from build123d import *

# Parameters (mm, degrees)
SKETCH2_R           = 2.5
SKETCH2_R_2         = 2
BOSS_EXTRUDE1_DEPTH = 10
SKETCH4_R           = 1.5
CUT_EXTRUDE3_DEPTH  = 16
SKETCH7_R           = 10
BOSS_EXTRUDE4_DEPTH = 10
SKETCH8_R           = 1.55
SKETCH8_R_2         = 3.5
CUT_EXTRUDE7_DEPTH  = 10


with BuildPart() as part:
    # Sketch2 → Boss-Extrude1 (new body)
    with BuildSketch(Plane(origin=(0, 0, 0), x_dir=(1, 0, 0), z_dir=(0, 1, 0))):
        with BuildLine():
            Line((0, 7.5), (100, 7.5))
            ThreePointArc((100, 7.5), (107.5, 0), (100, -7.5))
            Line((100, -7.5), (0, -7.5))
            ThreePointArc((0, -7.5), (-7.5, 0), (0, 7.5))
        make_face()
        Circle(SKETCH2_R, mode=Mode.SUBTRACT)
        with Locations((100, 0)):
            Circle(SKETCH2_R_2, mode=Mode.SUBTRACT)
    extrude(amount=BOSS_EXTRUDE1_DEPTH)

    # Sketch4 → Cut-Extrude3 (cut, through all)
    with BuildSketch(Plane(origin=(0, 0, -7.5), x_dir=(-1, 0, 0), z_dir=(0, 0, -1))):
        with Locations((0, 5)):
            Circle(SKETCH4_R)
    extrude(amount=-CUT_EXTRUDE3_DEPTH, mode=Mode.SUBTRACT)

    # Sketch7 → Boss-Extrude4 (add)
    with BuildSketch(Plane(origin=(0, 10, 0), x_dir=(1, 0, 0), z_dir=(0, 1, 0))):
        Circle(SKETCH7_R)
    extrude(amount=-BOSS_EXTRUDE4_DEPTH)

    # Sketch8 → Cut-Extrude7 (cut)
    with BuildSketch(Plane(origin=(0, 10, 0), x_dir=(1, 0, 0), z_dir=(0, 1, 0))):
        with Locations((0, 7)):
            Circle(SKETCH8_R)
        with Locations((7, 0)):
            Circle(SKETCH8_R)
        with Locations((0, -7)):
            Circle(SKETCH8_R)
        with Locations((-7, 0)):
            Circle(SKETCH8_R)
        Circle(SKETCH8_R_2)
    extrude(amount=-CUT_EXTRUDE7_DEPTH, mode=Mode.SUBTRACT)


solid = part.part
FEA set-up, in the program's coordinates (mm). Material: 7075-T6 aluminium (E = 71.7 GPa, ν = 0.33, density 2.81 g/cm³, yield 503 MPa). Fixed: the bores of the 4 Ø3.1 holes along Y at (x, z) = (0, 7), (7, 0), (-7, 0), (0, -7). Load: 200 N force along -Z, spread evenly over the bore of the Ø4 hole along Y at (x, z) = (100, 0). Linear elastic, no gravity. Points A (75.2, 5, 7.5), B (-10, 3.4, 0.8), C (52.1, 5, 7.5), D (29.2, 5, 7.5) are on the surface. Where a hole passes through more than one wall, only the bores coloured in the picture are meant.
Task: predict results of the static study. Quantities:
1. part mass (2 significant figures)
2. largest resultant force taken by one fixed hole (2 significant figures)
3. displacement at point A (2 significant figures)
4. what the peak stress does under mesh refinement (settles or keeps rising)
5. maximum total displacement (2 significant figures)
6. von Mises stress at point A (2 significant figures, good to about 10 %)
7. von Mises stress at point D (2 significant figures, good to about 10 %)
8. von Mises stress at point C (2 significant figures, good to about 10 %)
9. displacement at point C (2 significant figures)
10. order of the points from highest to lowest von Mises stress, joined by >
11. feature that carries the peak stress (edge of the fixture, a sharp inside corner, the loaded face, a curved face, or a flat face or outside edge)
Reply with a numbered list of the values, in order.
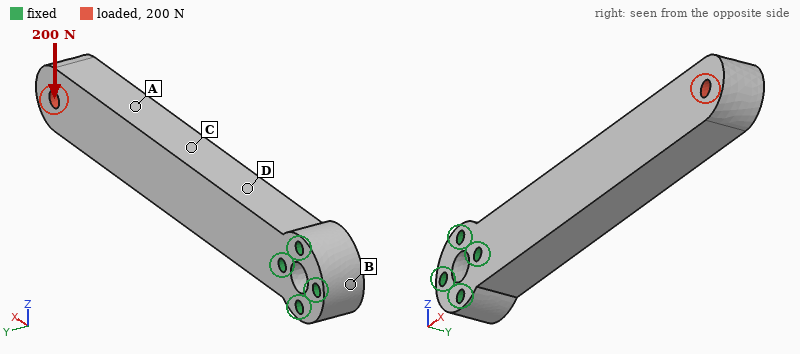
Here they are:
1. 47 g
2. 1.1 kN
3. 0.19 mm
4. keeps rising
5. 0.34 mm
6. 13 MPa
7. 38 MPa
8. 26 MPa
9. 0.10 mm
10. D > C > A > B
11. a sharp inside corner
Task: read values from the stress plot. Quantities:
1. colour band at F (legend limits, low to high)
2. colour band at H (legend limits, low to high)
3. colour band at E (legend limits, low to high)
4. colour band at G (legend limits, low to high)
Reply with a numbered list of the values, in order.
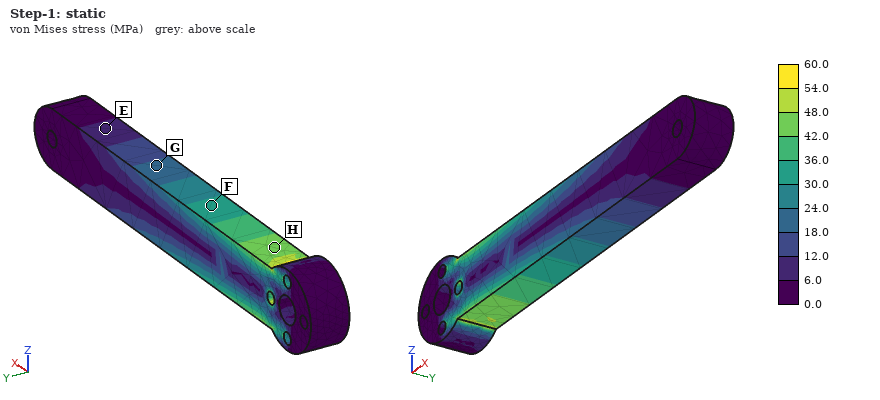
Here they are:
1. 30.0 to 36.0 MPa
2. 42.0 to 48.0 MPa
3. 6.0 to 12.0 MPa
4. 18.0 to 24.0 MPa
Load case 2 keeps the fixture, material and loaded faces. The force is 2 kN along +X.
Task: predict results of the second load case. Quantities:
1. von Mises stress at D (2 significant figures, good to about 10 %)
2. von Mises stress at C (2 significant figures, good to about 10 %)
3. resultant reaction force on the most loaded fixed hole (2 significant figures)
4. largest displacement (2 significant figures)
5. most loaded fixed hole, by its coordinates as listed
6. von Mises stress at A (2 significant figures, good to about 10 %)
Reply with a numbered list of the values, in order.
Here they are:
1. 13 MPa
2. 13 MPa
3. 1.3 kN
4. 19 µm
5. (7, 0)
6. 13 MPa
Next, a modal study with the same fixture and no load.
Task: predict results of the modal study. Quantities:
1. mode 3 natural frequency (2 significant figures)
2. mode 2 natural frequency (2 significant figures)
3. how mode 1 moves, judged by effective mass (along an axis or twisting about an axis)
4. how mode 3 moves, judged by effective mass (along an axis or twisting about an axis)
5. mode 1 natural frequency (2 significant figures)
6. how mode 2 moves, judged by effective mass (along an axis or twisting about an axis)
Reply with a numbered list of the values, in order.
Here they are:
1. 4900 Hz
2. 1200 Hz
3. along Y
4. along Y
5. 830 Hz
6. along Z
